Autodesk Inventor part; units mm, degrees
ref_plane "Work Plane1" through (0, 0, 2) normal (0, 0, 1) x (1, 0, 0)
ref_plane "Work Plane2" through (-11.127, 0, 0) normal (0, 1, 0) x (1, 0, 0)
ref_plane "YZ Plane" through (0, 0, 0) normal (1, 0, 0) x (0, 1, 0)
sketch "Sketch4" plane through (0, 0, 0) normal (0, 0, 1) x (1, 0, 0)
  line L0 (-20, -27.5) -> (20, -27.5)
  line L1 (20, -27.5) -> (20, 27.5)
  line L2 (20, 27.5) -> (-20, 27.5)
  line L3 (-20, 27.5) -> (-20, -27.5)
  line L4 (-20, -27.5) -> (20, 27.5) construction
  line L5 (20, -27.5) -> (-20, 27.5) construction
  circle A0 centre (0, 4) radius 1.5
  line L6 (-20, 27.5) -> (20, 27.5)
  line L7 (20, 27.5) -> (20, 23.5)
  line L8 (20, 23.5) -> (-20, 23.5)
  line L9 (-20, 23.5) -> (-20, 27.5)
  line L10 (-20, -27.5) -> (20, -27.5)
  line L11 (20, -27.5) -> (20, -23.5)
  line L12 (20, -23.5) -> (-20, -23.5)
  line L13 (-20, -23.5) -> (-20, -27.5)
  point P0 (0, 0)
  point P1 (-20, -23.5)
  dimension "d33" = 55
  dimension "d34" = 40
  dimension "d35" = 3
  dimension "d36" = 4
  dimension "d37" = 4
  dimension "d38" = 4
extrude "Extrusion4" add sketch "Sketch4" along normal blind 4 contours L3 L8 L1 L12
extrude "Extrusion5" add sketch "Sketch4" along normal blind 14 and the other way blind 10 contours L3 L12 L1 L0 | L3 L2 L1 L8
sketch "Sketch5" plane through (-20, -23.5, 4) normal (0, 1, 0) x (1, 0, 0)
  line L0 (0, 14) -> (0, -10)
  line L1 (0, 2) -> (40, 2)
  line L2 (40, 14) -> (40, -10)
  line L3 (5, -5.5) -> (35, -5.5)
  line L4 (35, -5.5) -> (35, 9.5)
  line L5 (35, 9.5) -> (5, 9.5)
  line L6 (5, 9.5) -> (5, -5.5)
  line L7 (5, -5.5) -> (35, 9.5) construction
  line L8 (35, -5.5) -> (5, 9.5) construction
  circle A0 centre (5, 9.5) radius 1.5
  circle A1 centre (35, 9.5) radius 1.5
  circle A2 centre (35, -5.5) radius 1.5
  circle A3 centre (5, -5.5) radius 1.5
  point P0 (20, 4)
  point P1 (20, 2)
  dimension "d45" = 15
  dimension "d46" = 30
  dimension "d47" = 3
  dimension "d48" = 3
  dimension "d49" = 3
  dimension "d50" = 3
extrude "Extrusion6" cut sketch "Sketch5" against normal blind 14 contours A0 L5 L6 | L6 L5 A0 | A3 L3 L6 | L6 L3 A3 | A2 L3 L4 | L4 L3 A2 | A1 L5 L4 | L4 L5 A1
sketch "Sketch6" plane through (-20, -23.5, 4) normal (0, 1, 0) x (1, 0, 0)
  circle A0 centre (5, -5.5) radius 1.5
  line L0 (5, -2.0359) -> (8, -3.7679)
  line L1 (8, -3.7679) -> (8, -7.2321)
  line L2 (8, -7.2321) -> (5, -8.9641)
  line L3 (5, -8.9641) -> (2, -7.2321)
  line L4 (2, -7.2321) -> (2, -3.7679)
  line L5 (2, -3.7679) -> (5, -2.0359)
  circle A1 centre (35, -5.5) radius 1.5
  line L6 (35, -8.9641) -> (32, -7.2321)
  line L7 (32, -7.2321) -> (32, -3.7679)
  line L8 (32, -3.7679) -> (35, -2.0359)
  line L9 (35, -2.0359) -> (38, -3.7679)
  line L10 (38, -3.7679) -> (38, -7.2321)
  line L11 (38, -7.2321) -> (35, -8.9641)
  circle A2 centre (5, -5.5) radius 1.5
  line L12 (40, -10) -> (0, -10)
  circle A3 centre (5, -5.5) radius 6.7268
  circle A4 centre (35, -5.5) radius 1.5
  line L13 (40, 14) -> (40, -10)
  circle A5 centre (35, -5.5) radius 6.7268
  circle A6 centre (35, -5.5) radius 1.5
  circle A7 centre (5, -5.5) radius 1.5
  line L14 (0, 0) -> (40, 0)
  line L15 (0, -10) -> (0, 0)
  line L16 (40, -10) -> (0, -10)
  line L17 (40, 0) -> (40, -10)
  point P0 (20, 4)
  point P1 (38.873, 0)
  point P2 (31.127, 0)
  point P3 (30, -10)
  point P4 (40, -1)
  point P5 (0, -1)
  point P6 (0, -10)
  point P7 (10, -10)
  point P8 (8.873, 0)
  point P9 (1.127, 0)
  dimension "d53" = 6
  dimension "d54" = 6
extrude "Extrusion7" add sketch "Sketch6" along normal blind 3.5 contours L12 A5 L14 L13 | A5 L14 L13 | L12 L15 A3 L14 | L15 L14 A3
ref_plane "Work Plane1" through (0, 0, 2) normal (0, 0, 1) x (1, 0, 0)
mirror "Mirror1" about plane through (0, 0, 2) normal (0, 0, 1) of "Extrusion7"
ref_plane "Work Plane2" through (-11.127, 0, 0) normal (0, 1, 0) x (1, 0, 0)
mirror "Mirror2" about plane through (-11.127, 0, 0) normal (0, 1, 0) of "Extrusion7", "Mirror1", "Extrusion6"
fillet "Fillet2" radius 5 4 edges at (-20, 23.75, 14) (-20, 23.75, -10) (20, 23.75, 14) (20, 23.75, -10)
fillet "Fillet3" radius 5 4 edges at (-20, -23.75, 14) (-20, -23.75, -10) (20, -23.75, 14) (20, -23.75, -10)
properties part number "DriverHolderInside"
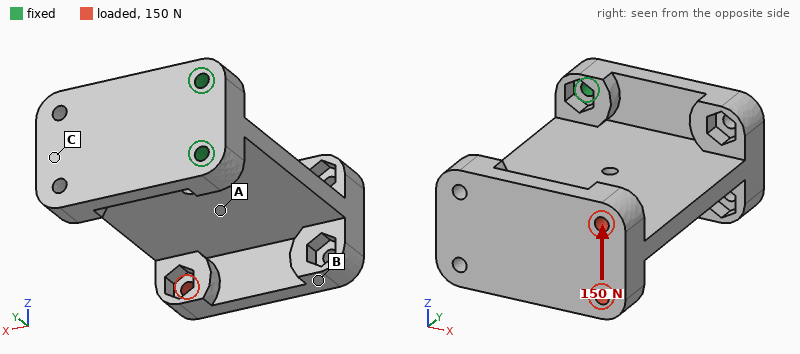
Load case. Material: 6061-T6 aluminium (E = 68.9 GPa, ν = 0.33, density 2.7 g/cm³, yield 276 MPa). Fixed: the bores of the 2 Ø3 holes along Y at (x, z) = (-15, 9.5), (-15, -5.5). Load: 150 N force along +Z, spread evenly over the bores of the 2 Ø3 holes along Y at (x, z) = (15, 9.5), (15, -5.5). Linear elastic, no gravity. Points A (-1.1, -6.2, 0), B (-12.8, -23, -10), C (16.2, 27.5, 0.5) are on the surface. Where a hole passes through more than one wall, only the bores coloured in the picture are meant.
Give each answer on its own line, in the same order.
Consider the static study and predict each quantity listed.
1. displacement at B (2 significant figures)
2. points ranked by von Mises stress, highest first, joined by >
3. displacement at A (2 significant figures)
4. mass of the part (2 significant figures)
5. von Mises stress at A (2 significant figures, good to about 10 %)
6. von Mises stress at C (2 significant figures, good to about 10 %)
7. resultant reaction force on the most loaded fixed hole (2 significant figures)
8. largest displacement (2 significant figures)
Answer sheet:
0.41 mm
A > C > B
0.22 mm
45 g
29 MPa
13 MPa
600 N
0.61 mm
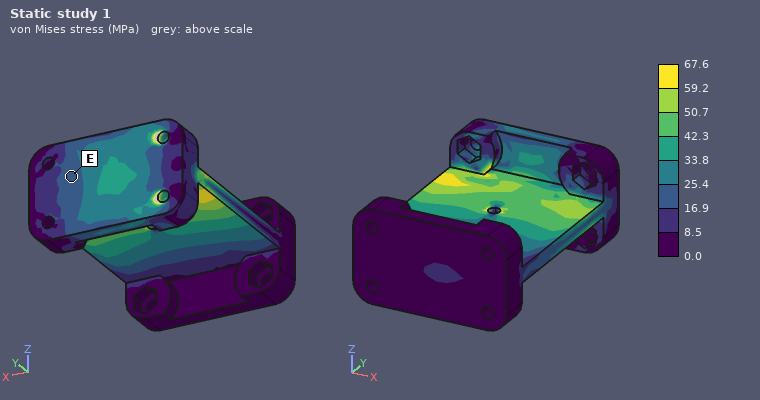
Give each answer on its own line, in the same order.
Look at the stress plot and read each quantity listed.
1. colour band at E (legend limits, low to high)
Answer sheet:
16.9 to 25.4 MPa
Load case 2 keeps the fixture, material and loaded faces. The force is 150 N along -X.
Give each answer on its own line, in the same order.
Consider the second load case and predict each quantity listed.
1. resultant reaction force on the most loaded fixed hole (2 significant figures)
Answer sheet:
86 N
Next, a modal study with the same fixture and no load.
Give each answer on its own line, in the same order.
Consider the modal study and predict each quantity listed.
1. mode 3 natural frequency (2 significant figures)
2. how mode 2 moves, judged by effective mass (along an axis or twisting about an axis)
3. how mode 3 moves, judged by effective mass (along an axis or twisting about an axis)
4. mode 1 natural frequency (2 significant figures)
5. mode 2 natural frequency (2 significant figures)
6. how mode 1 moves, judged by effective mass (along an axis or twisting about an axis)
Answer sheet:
2200 Hz
along X
twisting about Y
700 Hz
1100 Hz
along Z
